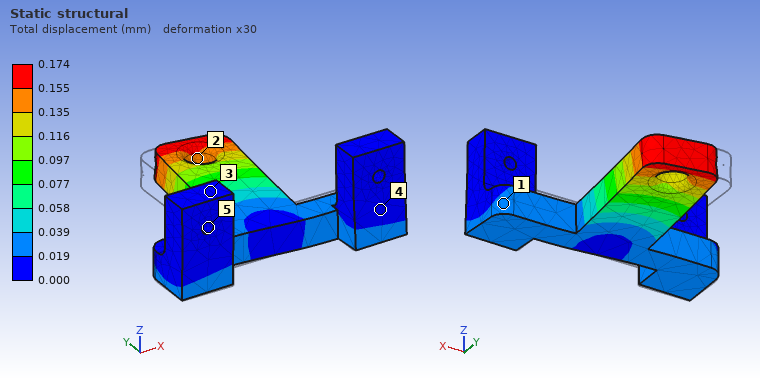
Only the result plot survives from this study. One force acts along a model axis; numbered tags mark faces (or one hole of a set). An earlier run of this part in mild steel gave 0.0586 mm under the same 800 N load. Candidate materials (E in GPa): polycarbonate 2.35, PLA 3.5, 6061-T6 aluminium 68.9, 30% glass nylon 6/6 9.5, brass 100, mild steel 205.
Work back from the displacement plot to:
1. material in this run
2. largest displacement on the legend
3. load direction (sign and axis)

6061-T6 aluminium
0.174 mm
+X
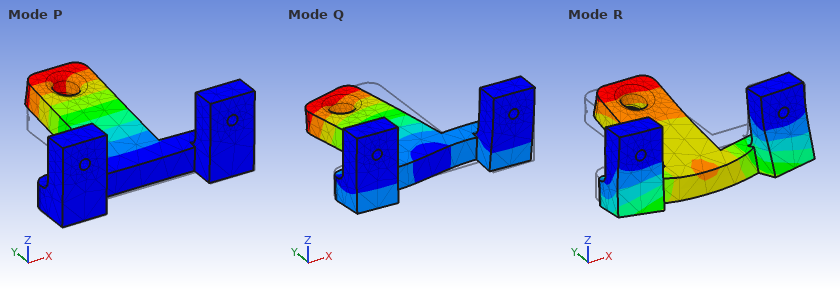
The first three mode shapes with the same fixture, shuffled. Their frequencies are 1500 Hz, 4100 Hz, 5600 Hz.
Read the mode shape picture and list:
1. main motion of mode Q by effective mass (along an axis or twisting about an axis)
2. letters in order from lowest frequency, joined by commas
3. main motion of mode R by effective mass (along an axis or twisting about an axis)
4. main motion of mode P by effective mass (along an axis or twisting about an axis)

along X
P, Q, R
along Y
along Z
